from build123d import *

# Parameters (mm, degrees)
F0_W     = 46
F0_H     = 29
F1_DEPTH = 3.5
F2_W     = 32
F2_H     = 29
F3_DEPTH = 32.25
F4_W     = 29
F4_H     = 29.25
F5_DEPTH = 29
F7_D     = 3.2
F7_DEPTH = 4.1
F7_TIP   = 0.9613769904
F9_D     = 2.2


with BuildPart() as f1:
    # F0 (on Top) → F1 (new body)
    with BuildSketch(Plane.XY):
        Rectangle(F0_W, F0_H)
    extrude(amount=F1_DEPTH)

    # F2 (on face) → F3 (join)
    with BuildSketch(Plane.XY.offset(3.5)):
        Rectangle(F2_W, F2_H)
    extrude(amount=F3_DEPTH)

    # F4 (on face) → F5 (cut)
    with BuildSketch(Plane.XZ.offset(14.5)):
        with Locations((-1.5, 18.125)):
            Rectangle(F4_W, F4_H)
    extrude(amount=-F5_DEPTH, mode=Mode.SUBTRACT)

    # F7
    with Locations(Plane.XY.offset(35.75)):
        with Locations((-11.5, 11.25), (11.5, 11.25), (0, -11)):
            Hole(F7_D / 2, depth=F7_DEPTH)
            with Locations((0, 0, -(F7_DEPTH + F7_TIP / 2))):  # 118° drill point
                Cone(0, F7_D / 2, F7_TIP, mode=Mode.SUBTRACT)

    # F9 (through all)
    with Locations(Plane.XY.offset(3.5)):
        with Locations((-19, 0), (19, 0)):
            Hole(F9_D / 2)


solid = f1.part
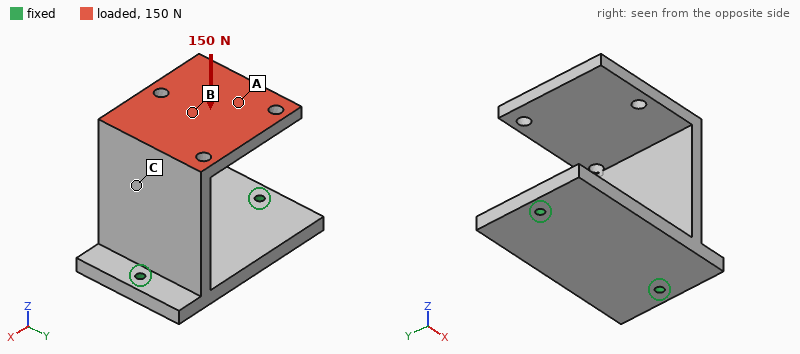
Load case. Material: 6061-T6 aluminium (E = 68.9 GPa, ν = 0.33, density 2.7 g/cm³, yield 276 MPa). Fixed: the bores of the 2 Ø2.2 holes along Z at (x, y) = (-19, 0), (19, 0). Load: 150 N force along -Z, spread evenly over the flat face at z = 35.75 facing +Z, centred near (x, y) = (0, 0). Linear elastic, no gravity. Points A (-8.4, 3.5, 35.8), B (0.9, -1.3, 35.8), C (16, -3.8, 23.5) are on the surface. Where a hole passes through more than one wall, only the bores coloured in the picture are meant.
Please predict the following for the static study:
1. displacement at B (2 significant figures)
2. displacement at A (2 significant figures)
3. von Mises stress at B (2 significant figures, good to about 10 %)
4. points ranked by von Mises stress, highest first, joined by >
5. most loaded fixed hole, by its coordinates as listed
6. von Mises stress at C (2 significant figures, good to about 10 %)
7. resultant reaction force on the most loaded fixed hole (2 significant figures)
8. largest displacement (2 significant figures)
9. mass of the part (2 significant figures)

0.39 mm
0.53 mm
14 MPa
C > B > A
(19, 0)
43 MPa
93 N
0.66 mm
27 g
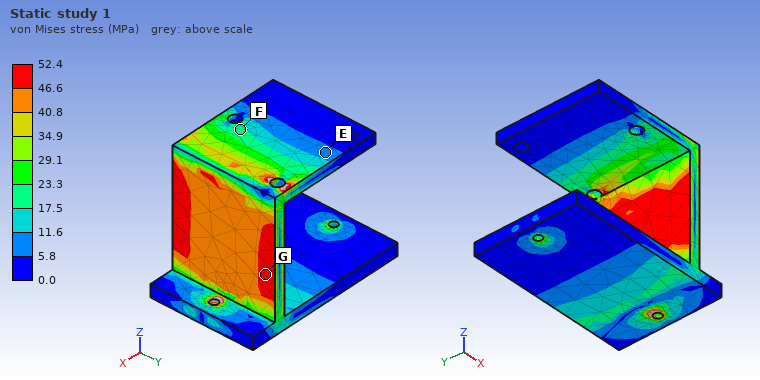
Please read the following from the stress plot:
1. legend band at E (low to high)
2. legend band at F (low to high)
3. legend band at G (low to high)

5.8 to 11.6 MPa
17.5 to 23.3 MPa
46.6 to 52.4 MPa
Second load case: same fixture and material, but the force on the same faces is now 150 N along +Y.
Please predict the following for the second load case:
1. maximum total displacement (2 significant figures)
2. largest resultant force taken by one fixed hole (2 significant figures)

0.36 mm
79 N
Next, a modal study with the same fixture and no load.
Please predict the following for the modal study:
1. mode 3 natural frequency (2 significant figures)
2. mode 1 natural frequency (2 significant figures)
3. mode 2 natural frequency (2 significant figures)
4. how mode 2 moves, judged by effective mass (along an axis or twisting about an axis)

2300 Hz
810 Hz
1300 Hz
along Y
